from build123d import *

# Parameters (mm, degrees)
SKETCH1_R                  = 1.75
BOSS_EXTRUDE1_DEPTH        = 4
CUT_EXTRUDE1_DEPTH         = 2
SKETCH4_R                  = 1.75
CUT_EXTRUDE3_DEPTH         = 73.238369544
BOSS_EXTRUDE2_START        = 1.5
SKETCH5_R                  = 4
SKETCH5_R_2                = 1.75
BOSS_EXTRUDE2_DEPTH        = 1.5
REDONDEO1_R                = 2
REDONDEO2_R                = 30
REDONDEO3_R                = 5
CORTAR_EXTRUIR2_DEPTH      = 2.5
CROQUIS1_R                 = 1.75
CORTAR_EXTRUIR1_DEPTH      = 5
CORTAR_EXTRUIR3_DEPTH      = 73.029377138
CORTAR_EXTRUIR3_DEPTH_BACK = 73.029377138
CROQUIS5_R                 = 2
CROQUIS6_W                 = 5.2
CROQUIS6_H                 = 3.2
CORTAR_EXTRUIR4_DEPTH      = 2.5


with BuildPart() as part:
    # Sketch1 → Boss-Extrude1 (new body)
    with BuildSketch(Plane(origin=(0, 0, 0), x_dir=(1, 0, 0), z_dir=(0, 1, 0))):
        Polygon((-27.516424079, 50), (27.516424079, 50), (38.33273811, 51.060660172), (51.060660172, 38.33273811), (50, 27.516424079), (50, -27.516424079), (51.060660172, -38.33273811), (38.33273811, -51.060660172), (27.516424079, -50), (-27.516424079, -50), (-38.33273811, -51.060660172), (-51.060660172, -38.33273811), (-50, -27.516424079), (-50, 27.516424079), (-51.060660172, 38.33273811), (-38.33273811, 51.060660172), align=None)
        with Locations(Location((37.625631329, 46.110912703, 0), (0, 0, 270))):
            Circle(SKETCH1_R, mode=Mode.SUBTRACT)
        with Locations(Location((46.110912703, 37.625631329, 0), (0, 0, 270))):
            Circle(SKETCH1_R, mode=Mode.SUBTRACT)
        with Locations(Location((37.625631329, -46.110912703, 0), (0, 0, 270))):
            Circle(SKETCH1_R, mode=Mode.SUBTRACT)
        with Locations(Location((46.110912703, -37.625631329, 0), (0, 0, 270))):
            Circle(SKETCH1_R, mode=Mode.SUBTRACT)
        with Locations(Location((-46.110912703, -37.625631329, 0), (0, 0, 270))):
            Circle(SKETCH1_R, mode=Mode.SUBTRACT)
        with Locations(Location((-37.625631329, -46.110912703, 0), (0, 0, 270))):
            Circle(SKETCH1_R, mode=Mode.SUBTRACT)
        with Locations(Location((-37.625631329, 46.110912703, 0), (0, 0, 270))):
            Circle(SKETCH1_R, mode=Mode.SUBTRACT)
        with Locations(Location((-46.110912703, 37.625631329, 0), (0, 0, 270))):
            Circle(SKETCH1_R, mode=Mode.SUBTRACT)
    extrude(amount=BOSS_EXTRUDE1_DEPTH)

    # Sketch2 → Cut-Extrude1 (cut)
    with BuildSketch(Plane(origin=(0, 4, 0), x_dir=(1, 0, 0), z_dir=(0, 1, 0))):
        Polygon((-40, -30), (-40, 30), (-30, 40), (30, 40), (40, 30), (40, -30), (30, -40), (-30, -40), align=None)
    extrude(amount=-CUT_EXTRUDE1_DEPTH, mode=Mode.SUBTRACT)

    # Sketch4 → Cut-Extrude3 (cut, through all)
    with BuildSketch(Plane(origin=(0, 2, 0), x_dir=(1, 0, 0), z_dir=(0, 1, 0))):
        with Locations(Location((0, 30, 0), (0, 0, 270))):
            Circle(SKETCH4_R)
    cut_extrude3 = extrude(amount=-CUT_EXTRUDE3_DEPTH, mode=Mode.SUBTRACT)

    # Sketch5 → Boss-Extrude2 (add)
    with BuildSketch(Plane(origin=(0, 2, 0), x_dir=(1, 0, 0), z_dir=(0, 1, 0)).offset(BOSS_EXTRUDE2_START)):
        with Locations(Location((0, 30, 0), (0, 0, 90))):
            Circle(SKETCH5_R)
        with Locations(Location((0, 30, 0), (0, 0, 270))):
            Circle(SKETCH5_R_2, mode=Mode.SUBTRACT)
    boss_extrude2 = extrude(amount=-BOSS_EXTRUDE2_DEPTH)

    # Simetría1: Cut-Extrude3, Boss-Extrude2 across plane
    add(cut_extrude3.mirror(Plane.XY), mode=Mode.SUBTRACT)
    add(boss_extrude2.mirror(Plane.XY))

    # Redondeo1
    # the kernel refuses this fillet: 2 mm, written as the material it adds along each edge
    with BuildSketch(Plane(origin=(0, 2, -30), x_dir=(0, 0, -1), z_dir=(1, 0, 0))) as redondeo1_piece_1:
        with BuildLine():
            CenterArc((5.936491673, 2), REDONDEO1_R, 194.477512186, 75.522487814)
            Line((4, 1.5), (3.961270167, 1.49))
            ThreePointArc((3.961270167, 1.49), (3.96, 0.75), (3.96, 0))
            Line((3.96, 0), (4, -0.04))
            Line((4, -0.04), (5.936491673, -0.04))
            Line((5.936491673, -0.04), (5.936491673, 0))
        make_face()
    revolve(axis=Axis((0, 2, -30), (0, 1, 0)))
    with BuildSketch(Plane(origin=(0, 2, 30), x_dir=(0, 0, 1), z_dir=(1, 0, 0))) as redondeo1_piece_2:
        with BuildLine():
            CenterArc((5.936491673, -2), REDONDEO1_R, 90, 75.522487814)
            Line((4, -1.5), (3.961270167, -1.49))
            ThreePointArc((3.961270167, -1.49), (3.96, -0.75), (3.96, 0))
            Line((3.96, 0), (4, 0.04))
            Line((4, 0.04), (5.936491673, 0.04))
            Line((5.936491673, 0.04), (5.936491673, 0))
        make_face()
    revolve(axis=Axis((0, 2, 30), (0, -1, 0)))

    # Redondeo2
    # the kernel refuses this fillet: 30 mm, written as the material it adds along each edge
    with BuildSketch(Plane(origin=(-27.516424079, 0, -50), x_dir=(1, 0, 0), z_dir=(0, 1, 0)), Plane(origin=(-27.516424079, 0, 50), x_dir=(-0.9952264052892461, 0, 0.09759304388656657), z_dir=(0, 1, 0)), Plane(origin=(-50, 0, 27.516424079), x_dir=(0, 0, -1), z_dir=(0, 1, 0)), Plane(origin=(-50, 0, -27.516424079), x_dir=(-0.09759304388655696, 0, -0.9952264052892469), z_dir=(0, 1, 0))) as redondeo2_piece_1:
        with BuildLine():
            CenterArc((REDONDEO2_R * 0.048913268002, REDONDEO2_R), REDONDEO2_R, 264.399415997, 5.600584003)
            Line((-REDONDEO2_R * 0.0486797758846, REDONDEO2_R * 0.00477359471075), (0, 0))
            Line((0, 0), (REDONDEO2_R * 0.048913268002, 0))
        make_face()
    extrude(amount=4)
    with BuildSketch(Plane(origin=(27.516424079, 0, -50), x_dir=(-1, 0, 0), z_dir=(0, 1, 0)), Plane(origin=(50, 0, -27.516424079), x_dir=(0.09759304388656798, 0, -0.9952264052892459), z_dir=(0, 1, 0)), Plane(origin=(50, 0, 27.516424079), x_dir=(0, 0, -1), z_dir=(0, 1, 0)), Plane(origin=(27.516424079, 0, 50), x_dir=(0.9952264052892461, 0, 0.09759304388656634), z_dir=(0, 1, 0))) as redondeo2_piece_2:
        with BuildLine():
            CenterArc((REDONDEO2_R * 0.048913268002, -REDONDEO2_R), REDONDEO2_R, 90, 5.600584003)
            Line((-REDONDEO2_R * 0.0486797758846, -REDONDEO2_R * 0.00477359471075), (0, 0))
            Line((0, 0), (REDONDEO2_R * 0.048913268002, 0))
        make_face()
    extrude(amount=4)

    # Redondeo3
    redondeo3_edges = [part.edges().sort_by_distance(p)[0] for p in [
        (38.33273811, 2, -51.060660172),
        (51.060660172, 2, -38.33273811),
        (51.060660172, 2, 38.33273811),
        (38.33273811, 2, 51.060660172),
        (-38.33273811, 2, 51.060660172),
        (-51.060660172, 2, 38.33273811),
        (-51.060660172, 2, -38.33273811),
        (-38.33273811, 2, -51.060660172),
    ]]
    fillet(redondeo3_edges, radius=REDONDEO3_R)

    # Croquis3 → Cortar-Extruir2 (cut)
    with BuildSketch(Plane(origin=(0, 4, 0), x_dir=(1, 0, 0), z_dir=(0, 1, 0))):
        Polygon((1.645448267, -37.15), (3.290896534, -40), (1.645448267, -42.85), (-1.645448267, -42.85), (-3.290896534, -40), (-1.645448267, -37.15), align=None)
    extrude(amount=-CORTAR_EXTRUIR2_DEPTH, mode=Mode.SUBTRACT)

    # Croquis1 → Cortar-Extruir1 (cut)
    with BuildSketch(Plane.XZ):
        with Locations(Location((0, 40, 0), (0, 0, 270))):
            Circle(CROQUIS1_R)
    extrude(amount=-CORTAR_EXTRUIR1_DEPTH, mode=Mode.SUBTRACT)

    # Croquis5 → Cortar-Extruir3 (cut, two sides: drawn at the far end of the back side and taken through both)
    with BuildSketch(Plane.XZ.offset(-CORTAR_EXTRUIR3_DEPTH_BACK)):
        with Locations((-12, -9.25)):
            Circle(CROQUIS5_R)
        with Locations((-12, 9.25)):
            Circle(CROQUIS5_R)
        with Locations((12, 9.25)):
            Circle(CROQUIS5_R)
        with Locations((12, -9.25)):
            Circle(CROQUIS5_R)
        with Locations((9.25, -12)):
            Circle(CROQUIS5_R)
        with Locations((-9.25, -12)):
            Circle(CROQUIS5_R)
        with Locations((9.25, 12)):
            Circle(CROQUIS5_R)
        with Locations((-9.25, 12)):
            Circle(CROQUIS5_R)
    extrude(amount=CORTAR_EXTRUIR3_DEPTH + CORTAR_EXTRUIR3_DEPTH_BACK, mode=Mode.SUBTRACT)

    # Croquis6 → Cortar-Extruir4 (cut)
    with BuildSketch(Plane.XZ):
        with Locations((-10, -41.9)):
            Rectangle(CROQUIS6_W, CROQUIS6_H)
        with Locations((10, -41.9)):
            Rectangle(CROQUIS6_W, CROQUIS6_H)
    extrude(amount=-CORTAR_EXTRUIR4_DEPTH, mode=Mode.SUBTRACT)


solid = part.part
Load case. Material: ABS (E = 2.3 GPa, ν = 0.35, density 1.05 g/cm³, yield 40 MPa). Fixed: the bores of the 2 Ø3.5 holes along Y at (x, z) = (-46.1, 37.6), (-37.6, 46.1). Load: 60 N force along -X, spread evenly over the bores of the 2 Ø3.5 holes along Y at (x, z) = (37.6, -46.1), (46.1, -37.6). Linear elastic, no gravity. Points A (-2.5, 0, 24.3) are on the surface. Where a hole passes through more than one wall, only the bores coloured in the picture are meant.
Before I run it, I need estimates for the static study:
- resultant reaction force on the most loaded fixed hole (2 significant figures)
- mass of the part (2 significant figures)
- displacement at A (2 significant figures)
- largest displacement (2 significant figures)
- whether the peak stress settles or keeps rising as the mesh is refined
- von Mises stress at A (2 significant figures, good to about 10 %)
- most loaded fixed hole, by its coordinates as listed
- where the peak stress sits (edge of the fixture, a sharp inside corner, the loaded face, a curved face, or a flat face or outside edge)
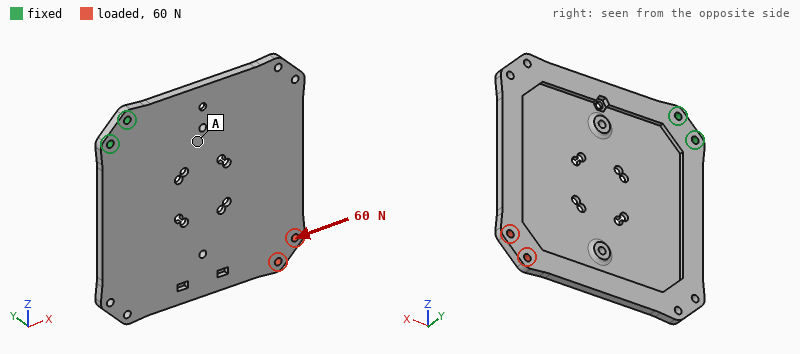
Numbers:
350 N
28 g
0.45 mm
1.5 mm
keeps rising
1.2 MPa
(-46.1, 37.6)
edge of the fixture
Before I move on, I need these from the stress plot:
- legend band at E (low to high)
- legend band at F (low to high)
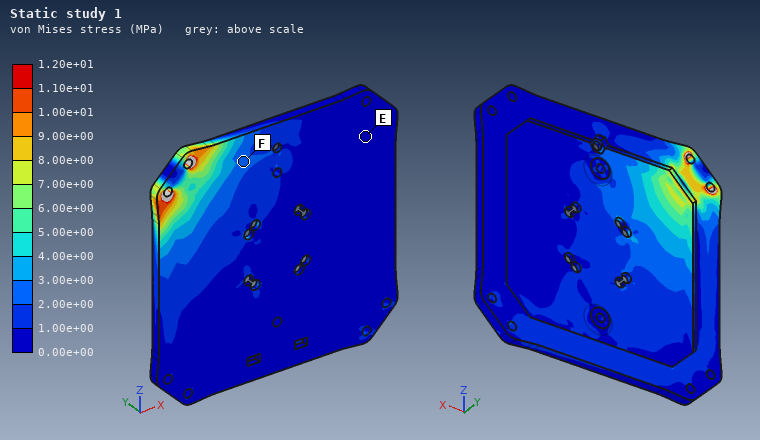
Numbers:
0.00e+00 to 1.00e+00 MPa
2.00e+00 to 3.00e+00 MPa
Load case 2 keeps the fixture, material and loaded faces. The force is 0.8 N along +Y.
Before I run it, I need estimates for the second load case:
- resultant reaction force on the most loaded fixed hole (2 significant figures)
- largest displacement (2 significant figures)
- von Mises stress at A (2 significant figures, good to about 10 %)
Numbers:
3.7 N
1.5 mm
0.42 MPa
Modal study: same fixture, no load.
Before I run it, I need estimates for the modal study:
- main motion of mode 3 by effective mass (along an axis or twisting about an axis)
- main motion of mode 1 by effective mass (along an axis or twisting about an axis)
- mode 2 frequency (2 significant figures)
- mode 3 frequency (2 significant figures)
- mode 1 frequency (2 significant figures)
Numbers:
along Y
along Y
100 Hz
220 Hz
49 Hz
